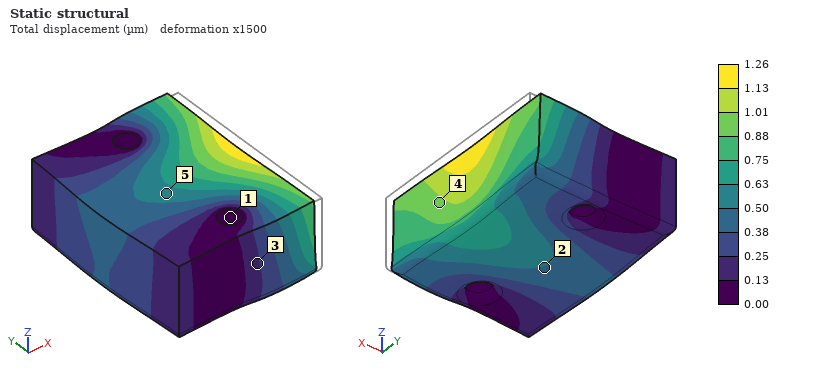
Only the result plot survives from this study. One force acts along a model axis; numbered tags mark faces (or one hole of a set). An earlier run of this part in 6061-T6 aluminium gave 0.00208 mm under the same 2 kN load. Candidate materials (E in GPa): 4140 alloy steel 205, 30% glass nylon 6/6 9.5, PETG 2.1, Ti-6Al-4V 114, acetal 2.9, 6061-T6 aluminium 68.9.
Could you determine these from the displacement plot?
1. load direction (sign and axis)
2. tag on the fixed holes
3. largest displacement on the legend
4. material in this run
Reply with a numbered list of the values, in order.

1. -X
2. 1
3. 1.26 µm
4. Ti-6Al-4V
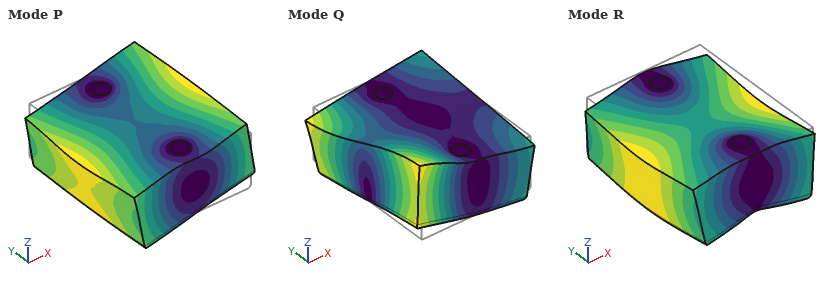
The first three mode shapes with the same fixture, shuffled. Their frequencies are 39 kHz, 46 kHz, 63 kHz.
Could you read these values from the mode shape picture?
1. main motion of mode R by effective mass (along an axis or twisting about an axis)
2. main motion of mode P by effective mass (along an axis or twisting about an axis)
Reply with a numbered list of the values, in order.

1. along Z
2. twisting about Y
